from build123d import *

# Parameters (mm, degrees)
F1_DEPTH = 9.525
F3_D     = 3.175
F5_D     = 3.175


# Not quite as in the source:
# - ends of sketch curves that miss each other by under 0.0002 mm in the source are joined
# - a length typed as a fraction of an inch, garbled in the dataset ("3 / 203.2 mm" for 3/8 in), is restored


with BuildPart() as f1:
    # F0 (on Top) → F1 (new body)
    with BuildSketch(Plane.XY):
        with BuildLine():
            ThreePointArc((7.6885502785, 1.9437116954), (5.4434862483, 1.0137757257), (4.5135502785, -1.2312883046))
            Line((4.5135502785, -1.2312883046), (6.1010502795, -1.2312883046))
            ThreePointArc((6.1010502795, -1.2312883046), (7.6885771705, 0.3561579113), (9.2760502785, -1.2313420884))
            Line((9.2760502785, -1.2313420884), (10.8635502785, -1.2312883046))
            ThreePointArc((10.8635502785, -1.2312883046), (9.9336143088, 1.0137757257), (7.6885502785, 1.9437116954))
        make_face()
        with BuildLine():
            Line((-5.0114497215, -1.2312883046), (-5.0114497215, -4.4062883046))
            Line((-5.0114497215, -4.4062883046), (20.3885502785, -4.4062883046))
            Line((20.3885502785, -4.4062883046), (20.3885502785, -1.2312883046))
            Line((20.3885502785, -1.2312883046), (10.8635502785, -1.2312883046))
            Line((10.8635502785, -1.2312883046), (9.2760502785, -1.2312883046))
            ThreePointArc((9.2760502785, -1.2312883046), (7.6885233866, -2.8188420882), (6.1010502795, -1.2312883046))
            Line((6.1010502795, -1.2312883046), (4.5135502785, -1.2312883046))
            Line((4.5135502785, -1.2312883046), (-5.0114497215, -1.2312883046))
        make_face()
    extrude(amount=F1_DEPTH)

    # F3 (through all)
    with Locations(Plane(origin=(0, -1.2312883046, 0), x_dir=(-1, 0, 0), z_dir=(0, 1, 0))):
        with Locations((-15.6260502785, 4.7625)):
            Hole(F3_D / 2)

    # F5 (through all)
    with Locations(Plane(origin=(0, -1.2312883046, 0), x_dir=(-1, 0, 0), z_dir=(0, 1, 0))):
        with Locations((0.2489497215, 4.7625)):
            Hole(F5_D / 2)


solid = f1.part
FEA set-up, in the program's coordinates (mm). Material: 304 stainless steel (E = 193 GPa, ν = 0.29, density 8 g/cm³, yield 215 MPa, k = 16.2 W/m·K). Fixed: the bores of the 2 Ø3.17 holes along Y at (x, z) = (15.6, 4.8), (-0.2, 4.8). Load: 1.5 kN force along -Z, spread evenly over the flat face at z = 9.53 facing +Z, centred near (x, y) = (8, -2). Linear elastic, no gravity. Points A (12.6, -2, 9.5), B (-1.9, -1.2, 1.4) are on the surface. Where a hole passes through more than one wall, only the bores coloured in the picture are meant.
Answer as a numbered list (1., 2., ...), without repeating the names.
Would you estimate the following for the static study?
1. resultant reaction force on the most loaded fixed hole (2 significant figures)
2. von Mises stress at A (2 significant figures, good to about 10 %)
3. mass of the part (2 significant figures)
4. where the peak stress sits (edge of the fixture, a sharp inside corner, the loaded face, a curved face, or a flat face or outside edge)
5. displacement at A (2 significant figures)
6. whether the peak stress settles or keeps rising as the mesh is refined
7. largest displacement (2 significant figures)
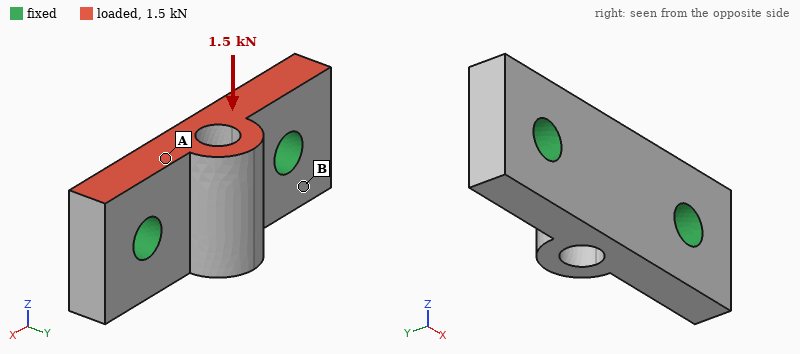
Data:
1. 750 N
2. 21 MPa
3. 6.3 g
4. edge of the fixture
5. 1.2 µm
6. keeps rising
7. 2.9 µm
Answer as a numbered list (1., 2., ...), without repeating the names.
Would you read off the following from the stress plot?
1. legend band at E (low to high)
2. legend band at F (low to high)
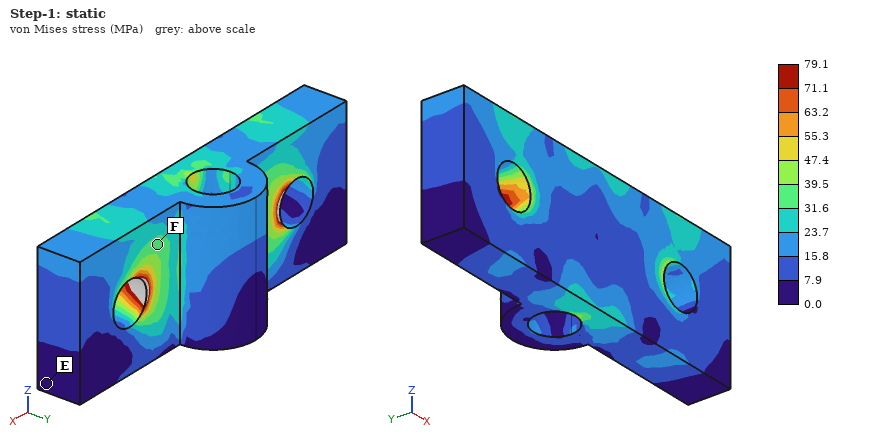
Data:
1. 0.0 to 7.9 MPa
2. 31.6 to 39.5 MPa
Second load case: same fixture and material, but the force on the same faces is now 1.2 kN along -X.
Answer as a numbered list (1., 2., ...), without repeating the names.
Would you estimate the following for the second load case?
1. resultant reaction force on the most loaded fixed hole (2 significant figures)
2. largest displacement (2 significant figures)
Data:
1. 650 N
2. 2.1 µm
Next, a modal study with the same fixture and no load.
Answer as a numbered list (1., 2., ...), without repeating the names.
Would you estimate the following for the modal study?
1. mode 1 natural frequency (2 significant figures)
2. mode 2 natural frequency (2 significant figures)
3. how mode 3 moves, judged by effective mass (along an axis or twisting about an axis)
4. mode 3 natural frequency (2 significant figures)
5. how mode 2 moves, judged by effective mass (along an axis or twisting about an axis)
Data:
1. 48 kHz
2. 54 kHz
3. along Z
4. 70 kHz
5. along Y
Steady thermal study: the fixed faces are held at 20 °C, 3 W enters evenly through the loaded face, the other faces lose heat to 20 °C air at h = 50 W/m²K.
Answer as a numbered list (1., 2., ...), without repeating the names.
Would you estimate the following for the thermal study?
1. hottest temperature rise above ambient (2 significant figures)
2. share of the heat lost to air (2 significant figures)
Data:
1. 15 K
2. 6.2 %
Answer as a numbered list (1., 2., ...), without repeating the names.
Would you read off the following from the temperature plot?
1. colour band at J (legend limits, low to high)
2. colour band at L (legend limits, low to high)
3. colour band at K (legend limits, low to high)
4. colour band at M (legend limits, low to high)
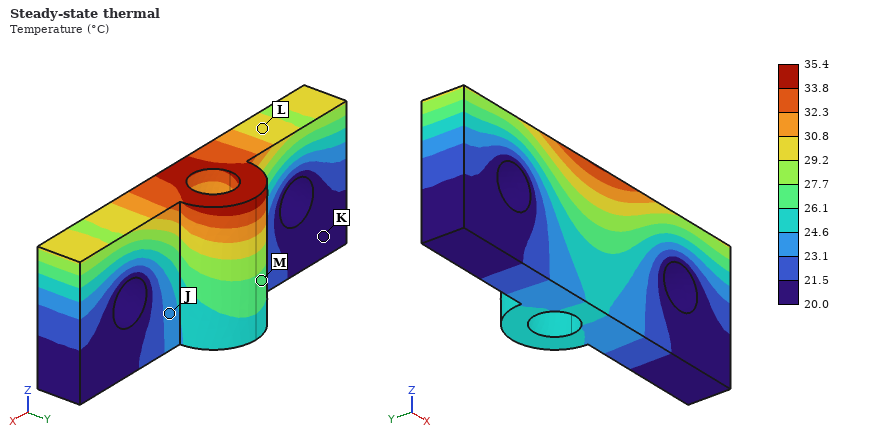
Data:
1. 23.1 to 24.6 °C
2. 29.2 to 30.8 °C
3. 20.0 to 21.5 °C
4. 26.1 to 27.7 °C
